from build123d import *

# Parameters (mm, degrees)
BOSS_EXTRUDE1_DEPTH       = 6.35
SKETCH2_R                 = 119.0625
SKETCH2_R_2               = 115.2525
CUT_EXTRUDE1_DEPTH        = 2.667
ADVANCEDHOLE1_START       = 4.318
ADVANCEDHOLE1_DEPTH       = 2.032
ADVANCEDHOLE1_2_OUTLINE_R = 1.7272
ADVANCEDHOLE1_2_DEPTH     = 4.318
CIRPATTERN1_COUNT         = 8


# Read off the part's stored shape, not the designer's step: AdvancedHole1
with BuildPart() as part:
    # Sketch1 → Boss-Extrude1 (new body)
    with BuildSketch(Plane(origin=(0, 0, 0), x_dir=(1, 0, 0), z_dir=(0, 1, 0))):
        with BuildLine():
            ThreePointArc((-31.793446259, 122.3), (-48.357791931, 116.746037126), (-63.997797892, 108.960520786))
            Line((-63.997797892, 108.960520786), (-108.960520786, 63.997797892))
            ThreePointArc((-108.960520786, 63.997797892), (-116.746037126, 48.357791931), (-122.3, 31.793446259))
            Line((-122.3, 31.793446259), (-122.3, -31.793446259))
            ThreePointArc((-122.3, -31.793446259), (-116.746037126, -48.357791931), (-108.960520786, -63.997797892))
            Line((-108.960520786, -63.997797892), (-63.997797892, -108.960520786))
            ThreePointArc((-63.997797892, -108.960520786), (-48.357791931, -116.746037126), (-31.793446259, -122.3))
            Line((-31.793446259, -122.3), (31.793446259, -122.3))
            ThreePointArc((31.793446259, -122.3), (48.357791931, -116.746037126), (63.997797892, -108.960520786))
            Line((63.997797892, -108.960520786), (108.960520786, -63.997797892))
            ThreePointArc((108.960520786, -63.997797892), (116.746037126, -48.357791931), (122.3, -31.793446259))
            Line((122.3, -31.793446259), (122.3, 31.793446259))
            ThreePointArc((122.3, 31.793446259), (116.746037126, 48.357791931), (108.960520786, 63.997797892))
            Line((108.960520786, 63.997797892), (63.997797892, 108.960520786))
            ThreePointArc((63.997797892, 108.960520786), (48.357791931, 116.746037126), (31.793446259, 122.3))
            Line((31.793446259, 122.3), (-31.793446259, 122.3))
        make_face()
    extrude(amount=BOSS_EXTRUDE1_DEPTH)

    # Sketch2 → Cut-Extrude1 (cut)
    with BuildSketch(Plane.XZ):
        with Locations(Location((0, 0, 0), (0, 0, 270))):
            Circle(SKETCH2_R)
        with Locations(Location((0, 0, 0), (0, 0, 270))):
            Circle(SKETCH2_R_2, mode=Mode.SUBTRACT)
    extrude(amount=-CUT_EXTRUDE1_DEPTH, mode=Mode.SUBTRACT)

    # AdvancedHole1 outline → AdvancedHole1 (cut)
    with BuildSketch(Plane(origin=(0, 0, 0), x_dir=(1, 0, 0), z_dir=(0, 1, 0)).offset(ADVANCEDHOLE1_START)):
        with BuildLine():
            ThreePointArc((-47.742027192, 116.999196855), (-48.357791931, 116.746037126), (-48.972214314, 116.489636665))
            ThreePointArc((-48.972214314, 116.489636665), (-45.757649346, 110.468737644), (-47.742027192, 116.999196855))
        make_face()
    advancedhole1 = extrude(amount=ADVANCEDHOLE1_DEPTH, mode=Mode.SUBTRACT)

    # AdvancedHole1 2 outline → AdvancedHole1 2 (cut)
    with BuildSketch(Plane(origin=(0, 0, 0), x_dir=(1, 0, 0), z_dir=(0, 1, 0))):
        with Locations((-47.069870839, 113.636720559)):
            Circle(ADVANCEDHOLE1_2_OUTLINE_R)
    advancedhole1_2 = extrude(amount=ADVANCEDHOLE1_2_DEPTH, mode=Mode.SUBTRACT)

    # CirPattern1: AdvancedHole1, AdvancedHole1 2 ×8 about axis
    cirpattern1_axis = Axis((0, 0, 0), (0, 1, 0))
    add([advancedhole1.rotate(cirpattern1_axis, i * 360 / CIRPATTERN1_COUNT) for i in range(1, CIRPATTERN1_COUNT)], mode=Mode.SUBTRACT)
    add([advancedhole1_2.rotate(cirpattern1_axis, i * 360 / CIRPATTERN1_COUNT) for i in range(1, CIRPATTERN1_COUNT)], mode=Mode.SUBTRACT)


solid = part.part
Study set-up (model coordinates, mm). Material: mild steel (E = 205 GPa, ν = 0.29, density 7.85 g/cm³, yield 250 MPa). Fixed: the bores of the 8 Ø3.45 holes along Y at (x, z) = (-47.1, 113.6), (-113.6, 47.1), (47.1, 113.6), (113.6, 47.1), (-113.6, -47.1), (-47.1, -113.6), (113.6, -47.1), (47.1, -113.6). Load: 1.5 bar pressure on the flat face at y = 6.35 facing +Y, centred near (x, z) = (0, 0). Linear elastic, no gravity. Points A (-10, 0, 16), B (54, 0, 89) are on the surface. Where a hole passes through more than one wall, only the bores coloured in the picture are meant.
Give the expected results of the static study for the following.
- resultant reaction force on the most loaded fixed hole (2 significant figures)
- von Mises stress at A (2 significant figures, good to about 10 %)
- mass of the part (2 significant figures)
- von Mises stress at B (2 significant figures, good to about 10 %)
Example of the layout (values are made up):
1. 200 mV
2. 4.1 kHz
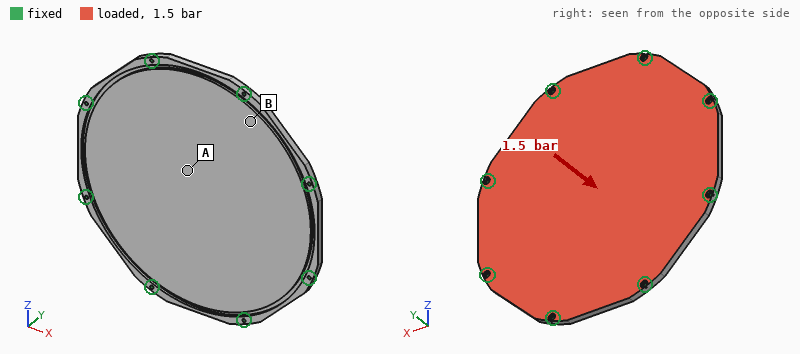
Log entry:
1. 920 N
2. 49 MPa
3. 2.4 kg
4. 25 MPa
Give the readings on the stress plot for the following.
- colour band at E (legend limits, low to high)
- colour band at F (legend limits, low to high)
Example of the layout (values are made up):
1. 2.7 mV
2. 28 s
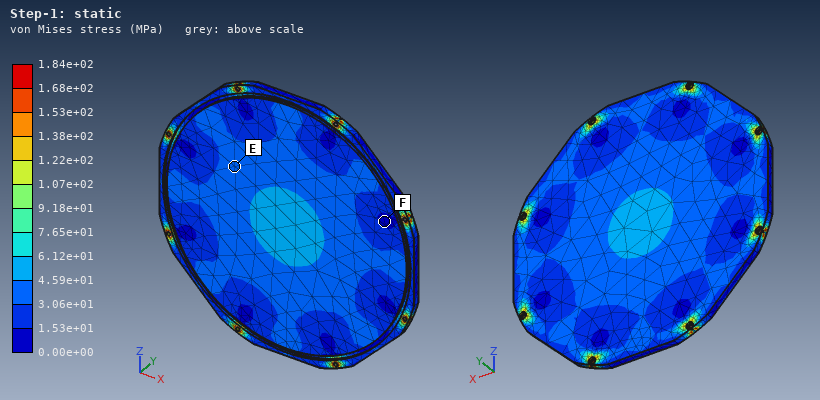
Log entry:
1. 3.06e+01 to 4.59e+01 MPa
2. 0.00e+00 to 1.53e+01 MPa
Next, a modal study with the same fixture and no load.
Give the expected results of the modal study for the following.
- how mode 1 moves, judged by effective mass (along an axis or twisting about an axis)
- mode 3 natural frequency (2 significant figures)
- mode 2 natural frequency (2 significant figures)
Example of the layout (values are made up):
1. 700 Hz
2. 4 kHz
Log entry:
1. along Y
2. 1500 Hz
3. 1500 Hz
